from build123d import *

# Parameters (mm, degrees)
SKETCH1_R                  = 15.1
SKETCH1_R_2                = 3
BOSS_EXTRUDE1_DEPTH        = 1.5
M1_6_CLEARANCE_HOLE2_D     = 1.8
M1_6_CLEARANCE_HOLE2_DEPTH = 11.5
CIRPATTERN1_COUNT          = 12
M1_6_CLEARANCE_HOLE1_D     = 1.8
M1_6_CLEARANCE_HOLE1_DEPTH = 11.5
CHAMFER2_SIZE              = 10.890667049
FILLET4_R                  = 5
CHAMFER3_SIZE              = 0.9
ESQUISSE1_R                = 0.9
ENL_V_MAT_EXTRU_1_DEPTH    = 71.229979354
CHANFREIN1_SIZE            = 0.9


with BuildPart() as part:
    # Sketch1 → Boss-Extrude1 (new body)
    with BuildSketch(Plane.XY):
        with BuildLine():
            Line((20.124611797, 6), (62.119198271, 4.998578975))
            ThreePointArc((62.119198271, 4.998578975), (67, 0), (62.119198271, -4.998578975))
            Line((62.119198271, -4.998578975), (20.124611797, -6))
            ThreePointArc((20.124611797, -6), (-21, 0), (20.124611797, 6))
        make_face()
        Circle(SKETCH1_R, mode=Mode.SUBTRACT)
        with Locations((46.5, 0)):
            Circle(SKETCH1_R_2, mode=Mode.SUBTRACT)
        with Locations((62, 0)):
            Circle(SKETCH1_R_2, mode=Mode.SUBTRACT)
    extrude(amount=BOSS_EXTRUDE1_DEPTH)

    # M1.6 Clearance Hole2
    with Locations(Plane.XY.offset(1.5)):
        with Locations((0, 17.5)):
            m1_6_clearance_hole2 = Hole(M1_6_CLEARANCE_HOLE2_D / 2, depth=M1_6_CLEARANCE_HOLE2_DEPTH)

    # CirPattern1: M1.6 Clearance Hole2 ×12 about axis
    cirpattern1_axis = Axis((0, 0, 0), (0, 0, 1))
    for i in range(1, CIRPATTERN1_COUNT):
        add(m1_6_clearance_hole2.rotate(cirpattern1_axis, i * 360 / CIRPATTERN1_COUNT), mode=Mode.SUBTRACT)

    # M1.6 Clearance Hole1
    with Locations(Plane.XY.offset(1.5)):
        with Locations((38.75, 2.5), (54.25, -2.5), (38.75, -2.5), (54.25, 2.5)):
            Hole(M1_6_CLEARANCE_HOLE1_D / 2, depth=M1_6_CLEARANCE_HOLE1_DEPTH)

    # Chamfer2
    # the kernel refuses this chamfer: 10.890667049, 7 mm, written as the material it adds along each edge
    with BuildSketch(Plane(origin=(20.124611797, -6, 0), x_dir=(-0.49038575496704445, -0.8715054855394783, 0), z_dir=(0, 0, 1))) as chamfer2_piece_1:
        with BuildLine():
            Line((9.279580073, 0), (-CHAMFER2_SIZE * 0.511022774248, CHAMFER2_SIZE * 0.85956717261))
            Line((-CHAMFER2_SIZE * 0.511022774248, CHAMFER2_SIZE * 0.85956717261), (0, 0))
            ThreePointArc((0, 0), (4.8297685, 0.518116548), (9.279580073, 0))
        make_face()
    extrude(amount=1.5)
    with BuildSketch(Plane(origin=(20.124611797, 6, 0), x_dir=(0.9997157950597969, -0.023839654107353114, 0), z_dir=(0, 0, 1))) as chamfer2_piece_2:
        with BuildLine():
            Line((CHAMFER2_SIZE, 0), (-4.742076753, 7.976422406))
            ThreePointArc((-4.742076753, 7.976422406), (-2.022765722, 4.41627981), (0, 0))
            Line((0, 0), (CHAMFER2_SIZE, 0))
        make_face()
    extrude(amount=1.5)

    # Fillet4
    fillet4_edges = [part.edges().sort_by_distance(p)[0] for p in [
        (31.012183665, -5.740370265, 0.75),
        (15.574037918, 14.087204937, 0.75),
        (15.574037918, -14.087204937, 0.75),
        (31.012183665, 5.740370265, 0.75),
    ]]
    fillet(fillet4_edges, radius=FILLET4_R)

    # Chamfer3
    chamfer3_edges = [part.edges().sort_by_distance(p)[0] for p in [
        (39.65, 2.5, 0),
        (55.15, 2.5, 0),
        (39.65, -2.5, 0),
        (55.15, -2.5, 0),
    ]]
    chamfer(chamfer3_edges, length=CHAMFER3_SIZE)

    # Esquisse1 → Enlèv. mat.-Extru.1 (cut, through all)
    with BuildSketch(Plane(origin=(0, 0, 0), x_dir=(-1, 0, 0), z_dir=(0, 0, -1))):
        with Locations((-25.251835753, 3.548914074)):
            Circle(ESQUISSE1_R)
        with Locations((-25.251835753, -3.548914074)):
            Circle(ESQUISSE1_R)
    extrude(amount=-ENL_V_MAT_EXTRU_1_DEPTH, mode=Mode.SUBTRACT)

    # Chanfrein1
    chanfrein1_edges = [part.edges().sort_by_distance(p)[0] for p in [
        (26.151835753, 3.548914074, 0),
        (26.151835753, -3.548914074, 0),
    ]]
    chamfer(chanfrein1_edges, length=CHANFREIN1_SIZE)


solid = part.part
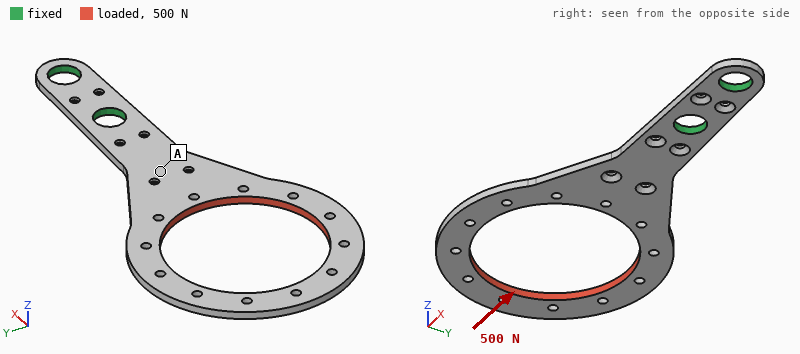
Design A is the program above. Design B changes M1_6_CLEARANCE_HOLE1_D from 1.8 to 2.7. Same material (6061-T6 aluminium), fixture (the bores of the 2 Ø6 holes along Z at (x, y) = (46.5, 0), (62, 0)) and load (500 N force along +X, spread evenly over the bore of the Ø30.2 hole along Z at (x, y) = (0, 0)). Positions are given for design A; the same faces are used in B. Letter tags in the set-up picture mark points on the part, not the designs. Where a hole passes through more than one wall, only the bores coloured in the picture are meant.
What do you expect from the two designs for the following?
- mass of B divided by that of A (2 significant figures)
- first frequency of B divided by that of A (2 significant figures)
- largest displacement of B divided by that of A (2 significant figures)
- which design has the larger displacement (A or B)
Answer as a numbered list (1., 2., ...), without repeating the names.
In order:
1. 0.99
2. 0.94
3. 1.5
4. B
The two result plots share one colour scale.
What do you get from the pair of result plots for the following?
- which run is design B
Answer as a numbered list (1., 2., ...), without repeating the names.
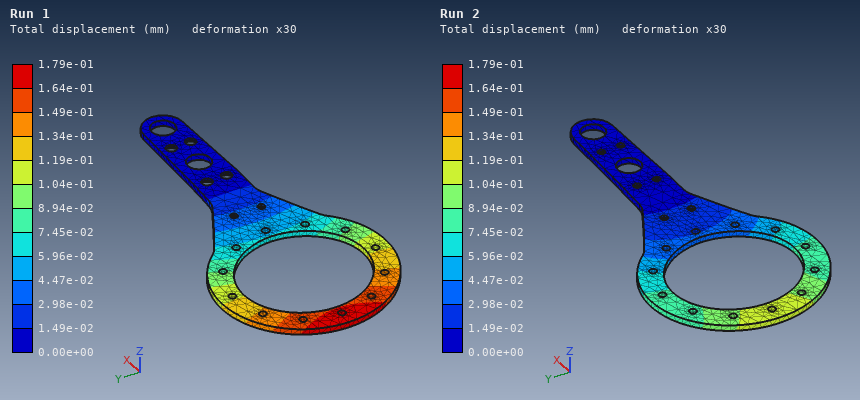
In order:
1. Run 1
